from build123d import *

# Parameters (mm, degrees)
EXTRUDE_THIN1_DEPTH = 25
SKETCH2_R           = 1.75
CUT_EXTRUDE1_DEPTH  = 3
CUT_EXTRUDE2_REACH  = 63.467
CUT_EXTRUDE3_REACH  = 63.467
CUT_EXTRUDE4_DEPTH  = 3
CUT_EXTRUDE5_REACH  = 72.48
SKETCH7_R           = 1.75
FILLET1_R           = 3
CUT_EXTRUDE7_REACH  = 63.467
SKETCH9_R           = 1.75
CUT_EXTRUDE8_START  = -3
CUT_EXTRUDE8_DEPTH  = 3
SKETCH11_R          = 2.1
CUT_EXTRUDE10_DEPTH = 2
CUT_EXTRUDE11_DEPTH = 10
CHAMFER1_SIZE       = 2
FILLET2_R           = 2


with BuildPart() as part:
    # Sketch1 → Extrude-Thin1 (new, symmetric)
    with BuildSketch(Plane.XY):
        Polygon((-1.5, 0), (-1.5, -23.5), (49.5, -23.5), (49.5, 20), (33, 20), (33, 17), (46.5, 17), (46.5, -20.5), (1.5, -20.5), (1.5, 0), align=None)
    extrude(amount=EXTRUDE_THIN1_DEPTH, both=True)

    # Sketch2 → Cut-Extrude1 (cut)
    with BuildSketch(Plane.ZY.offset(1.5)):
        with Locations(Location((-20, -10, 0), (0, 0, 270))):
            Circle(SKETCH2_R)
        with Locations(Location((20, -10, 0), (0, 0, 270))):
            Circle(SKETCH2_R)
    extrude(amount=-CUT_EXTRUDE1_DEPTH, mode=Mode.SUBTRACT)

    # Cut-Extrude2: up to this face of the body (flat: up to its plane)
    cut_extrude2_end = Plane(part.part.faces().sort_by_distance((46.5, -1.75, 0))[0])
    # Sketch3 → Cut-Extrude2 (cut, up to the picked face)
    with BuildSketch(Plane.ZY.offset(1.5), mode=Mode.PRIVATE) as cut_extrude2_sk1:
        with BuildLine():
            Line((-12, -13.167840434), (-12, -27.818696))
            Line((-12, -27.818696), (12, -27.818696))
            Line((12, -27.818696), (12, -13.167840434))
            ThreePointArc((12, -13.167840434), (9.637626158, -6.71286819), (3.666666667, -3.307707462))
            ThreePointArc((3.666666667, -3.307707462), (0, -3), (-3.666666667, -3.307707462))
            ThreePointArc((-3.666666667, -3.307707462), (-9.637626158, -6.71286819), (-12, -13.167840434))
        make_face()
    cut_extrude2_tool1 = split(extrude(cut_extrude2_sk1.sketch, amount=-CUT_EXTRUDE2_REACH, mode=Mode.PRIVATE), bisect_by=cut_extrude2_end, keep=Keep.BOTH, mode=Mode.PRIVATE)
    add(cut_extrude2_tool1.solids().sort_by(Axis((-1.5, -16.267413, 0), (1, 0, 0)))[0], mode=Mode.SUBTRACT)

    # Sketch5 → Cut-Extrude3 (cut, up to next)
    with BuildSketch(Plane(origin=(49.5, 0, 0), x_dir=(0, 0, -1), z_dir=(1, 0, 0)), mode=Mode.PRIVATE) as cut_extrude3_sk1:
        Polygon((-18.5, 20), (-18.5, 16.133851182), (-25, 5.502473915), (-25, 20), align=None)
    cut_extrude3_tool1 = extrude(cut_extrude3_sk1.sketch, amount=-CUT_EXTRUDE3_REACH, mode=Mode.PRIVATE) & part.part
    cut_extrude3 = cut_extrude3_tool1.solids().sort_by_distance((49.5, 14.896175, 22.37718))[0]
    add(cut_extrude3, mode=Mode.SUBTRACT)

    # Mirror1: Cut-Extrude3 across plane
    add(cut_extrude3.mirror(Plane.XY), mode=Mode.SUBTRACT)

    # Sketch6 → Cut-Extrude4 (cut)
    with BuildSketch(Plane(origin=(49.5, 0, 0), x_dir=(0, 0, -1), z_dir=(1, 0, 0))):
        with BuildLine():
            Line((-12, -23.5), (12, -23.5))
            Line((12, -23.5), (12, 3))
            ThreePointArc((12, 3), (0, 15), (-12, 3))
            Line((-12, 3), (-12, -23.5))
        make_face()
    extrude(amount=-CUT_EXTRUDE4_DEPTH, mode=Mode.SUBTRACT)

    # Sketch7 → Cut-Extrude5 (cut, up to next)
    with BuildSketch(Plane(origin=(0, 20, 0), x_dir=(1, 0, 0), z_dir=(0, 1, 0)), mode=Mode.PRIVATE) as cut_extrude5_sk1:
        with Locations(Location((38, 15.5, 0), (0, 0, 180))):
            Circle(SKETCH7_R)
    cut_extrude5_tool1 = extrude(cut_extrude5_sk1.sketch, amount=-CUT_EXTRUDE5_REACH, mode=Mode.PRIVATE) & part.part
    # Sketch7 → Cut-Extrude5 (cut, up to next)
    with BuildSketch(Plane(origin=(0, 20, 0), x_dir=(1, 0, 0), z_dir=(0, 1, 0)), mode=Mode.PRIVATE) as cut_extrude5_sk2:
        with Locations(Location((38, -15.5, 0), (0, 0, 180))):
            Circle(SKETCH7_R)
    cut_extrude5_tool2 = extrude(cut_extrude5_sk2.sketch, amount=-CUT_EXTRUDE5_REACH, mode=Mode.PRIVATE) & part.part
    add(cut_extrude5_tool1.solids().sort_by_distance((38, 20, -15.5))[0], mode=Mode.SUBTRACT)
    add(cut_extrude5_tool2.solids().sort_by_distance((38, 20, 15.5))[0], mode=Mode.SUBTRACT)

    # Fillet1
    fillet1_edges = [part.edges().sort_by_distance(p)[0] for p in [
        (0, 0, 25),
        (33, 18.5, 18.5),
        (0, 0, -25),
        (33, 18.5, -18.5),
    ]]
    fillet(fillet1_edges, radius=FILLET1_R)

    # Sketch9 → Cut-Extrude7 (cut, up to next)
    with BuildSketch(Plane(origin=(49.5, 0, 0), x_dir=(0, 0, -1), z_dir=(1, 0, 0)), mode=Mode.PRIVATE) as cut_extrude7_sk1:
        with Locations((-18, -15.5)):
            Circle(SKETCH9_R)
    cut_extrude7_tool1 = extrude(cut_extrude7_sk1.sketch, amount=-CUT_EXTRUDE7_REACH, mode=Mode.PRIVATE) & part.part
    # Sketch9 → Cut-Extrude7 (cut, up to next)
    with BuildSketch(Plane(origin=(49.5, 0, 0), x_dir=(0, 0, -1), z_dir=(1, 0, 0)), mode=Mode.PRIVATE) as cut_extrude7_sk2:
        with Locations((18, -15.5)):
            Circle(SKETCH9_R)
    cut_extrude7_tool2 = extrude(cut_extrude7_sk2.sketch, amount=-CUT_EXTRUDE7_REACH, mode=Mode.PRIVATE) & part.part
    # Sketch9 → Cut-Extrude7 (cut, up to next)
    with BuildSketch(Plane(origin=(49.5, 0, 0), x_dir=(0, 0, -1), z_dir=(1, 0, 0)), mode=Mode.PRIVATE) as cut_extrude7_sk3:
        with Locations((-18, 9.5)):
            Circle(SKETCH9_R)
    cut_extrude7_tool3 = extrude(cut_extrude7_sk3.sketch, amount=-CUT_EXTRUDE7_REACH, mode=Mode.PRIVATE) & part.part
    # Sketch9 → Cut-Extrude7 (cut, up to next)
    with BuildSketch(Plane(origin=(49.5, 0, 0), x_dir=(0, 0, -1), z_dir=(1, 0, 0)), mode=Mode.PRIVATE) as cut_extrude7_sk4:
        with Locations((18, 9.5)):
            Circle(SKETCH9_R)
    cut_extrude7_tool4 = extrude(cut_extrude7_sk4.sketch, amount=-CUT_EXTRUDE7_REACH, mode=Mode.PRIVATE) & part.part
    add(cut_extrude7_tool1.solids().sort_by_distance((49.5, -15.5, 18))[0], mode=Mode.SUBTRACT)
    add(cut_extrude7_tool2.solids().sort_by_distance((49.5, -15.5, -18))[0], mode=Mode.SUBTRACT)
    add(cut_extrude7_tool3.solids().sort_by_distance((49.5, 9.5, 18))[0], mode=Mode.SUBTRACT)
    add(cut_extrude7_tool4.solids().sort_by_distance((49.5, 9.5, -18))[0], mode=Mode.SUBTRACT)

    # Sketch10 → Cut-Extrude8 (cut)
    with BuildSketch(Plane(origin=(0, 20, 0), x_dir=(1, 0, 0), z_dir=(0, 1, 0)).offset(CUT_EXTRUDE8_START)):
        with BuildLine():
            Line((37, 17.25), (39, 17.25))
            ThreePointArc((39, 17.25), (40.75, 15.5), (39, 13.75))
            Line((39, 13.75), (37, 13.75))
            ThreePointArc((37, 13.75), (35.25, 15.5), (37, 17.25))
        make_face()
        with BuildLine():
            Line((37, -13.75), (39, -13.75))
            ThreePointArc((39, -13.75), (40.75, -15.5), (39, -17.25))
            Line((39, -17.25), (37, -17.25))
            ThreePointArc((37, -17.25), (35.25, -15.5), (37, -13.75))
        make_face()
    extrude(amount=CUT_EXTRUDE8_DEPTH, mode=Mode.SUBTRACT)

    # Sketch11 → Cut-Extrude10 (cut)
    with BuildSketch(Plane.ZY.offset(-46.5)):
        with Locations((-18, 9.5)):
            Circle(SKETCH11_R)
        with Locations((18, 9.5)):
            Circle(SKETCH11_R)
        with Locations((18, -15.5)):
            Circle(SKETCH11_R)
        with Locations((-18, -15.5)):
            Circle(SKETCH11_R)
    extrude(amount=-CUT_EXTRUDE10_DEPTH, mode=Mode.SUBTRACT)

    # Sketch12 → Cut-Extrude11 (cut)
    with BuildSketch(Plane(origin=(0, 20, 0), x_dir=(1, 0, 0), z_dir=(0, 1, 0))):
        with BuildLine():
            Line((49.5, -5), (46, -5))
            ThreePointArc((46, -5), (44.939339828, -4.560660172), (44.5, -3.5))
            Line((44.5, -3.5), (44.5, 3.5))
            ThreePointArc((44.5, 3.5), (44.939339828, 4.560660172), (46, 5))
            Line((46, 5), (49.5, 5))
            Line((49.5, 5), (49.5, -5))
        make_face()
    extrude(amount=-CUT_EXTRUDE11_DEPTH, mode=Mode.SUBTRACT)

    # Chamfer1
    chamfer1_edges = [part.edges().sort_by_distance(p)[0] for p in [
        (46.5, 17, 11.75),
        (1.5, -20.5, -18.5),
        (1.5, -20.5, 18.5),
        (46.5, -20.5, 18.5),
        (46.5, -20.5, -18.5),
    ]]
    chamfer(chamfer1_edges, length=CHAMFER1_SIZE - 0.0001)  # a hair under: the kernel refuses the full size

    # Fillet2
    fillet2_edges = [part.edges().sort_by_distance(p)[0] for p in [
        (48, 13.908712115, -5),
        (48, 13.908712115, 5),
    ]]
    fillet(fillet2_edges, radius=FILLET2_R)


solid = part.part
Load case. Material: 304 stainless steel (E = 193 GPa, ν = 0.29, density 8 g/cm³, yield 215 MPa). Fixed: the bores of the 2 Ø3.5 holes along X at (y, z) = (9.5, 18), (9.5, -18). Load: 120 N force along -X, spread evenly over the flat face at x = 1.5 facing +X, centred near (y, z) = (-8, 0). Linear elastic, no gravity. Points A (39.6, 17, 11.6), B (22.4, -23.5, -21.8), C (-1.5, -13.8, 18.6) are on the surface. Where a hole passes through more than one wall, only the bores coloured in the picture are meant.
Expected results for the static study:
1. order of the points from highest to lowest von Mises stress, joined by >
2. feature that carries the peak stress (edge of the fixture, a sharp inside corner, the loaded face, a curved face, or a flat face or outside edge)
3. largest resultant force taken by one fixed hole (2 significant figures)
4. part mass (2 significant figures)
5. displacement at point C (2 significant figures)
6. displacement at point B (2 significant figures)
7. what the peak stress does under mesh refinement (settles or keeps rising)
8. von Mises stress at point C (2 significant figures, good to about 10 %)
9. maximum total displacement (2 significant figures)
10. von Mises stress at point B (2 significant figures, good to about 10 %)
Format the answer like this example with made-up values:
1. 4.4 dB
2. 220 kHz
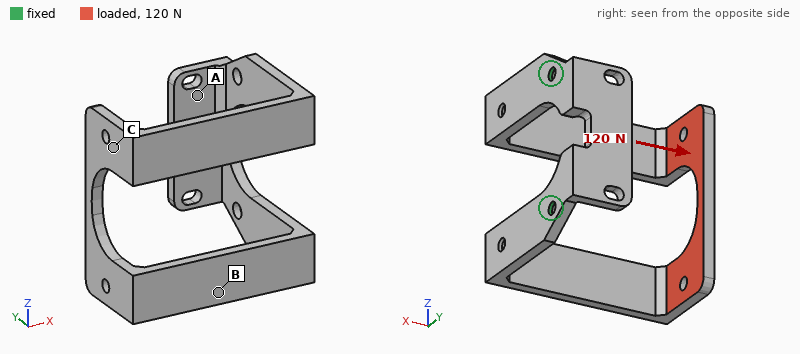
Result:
1. B > C > A
2. edge of the fixture
3. 60 N
4. 83 g
5. 0.14 mm
6. 0.058 mm
7. keeps rising
8. 18 MPa
9. 0.21 mm
10. 42 MPa
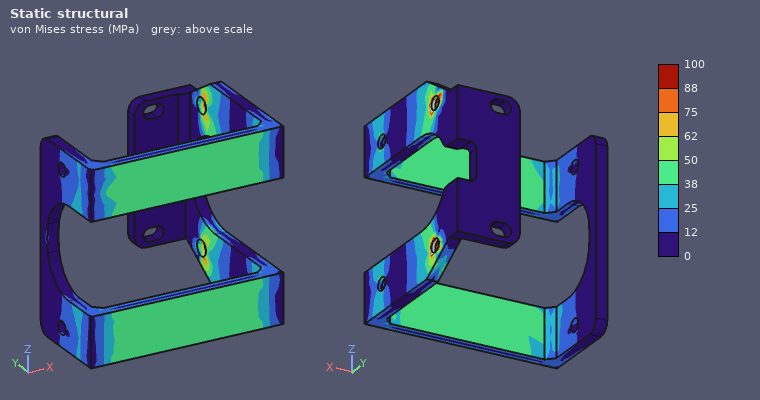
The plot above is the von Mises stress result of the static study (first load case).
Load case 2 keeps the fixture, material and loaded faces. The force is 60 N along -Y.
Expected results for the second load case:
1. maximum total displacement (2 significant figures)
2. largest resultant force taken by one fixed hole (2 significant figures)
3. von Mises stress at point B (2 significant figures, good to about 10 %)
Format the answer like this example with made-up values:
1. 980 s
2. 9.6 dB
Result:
1. 0.64 mm
2. 30 N
3. 32 MPa
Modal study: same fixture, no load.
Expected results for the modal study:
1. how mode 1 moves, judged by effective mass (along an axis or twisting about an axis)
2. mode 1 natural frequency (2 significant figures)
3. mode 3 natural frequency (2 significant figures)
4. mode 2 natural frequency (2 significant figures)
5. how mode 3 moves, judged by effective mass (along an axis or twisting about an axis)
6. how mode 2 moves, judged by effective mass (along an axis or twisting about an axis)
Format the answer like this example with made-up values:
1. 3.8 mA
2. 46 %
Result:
1. along Y
2. 290 Hz
3. 870 Hz
4. 480 Hz
5. along X
6. along Z
